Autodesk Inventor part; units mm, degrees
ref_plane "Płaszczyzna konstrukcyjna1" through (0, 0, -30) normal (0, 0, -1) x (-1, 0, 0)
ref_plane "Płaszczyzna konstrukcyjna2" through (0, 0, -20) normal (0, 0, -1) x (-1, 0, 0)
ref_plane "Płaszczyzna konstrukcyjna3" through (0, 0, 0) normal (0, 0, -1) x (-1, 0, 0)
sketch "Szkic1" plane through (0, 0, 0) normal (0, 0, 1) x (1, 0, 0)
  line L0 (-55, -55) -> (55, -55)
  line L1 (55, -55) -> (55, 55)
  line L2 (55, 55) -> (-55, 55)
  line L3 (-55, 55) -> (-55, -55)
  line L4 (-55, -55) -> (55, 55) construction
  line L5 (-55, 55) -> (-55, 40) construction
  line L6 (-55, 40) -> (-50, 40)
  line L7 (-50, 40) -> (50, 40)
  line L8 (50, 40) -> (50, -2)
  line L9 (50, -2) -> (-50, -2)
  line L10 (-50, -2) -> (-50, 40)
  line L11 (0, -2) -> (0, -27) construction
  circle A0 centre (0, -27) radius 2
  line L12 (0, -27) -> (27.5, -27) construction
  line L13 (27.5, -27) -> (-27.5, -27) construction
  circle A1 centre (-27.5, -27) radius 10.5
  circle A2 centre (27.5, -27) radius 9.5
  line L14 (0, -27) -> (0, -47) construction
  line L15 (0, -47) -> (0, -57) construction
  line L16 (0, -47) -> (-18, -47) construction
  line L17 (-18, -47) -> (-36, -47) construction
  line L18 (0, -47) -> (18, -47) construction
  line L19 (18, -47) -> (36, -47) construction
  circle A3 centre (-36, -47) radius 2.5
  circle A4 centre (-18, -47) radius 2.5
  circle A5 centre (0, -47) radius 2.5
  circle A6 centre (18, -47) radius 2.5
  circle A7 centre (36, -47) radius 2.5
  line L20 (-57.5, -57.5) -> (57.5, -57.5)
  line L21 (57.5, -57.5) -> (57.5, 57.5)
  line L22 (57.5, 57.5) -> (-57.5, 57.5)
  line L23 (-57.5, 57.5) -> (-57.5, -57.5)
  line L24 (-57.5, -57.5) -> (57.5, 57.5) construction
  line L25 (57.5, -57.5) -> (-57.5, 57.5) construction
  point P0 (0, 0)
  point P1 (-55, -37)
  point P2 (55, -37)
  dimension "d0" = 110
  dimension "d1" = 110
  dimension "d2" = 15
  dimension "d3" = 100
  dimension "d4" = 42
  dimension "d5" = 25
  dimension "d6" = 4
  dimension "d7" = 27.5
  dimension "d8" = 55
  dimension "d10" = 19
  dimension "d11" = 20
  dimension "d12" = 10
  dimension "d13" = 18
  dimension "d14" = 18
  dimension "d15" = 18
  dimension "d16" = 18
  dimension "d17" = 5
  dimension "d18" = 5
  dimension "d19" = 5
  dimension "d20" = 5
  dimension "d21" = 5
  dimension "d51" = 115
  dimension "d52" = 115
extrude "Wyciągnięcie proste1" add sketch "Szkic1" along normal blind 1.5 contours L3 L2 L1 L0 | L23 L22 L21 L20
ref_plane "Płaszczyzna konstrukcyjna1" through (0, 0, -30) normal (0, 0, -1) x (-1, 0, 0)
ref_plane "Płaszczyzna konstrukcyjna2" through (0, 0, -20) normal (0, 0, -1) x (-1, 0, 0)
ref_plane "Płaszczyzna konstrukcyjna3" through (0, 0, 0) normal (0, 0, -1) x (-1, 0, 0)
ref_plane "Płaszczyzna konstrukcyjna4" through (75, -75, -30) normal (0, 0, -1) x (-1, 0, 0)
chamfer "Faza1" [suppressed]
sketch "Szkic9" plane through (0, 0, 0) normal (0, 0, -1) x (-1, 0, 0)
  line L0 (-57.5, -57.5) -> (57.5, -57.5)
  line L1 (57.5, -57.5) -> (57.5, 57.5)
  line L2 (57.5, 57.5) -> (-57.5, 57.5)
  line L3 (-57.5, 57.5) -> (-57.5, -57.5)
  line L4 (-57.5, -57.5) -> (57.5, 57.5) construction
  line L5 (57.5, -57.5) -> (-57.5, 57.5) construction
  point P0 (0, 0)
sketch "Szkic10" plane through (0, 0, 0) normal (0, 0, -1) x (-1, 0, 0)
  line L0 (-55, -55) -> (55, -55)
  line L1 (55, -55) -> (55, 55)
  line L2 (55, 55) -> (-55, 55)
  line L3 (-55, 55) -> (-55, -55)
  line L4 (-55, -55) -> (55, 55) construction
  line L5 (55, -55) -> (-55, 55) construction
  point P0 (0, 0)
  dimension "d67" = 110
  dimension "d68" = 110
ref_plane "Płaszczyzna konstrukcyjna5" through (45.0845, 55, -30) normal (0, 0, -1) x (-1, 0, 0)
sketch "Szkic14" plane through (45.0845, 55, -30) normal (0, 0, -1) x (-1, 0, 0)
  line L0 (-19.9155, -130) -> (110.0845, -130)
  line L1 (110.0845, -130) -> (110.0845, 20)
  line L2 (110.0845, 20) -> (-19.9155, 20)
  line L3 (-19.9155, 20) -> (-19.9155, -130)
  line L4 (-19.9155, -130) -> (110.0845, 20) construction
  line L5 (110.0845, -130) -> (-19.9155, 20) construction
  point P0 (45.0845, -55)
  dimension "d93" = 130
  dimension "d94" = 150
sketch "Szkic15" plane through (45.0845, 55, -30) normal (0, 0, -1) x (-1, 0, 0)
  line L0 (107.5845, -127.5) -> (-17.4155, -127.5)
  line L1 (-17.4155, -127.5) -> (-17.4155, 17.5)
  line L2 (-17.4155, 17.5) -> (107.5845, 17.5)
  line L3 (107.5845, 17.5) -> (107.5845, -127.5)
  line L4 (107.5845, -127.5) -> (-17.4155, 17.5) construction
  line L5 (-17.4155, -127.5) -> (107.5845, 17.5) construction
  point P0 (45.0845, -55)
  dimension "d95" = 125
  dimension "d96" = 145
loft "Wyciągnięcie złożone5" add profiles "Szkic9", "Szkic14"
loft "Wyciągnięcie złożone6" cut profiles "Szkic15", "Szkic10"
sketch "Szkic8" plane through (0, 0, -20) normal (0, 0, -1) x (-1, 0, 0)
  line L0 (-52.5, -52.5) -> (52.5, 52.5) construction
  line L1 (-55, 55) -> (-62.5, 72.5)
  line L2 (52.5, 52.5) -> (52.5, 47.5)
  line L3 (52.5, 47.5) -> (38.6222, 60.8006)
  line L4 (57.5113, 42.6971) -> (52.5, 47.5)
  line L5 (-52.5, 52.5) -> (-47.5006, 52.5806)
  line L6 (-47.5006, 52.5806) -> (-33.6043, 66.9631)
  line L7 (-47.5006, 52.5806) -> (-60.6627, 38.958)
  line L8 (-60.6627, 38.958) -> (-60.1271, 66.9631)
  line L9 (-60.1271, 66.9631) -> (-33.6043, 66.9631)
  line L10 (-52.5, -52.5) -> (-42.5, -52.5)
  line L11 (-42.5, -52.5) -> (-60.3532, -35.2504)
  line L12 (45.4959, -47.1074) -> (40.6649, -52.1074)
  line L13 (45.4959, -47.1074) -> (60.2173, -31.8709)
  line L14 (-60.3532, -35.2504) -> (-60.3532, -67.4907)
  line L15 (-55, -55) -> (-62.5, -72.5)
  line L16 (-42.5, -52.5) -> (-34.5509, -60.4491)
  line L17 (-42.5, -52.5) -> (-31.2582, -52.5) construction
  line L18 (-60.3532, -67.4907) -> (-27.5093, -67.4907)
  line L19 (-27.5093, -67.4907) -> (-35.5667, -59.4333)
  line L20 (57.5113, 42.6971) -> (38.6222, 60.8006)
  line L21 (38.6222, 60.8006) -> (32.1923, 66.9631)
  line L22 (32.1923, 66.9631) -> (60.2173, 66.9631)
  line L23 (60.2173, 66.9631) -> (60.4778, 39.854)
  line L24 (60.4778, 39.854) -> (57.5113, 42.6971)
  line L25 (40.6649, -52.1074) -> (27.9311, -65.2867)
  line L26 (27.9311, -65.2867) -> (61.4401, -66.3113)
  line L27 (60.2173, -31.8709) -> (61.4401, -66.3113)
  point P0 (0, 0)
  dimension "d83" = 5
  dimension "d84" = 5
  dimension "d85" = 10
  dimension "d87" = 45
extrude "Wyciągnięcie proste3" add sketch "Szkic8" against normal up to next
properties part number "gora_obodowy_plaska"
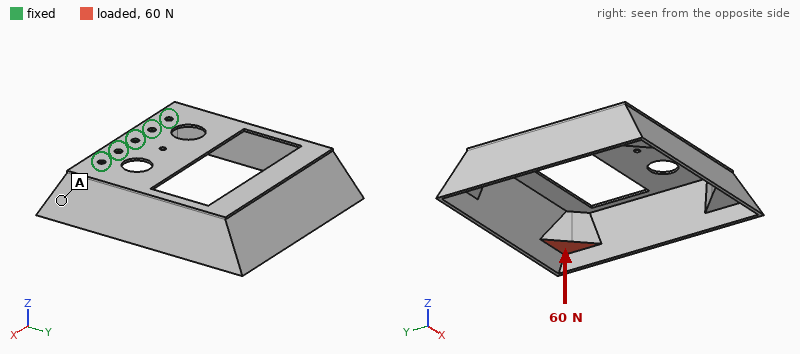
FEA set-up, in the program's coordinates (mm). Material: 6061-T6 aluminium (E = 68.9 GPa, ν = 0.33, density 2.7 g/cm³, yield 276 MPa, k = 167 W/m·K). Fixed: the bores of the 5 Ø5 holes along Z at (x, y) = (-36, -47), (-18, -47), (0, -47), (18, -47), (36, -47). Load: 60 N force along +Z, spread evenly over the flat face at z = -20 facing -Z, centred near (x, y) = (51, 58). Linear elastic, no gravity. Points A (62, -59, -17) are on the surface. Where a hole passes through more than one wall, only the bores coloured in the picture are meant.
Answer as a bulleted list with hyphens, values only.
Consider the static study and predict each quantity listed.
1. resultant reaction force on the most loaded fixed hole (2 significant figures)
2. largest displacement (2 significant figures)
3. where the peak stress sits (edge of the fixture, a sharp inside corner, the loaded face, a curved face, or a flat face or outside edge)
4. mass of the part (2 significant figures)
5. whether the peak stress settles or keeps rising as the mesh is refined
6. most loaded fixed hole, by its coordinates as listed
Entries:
- 190 N
- 2.0 mm
- edge of the fixture
- 190 g
- keeps rising
- (36, -47)
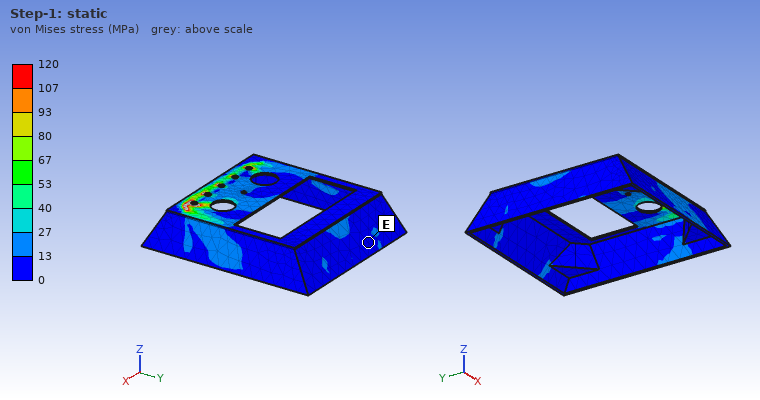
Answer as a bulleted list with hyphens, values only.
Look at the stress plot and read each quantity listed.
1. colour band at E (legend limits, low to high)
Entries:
- 0 to 13 MPa
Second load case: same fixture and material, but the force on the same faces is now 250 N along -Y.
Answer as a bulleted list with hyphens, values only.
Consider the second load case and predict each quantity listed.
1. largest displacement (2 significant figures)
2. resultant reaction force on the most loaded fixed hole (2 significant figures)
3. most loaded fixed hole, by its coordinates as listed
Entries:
- 1.7 mm
- 380 N
- (36, -47)
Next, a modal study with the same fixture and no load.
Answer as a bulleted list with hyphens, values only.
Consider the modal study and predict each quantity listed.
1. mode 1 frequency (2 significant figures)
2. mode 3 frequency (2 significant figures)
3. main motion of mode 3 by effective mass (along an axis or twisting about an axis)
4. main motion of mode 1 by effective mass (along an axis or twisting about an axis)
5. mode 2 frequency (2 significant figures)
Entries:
- 130 Hz
- 610 Hz
- along X
- along Z
- 240 Hz
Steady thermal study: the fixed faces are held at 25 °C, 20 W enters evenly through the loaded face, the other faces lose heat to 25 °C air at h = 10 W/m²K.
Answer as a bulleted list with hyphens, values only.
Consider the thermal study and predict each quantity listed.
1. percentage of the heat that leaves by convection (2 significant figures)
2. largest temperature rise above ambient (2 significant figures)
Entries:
- 48 %
- 60 K
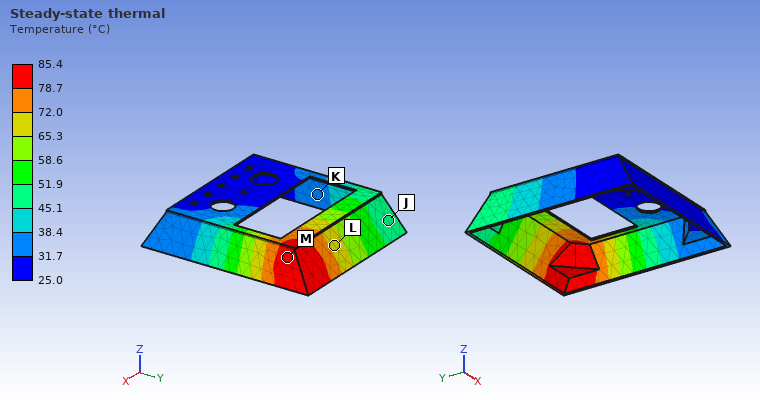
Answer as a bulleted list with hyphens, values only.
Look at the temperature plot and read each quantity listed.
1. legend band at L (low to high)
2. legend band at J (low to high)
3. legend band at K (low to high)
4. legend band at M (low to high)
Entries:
- 65.3 to 72.0 °C
- 45.1 to 51.9 °C
- 31.7 to 38.4 °C
- 78.7 to 85.4 °C
